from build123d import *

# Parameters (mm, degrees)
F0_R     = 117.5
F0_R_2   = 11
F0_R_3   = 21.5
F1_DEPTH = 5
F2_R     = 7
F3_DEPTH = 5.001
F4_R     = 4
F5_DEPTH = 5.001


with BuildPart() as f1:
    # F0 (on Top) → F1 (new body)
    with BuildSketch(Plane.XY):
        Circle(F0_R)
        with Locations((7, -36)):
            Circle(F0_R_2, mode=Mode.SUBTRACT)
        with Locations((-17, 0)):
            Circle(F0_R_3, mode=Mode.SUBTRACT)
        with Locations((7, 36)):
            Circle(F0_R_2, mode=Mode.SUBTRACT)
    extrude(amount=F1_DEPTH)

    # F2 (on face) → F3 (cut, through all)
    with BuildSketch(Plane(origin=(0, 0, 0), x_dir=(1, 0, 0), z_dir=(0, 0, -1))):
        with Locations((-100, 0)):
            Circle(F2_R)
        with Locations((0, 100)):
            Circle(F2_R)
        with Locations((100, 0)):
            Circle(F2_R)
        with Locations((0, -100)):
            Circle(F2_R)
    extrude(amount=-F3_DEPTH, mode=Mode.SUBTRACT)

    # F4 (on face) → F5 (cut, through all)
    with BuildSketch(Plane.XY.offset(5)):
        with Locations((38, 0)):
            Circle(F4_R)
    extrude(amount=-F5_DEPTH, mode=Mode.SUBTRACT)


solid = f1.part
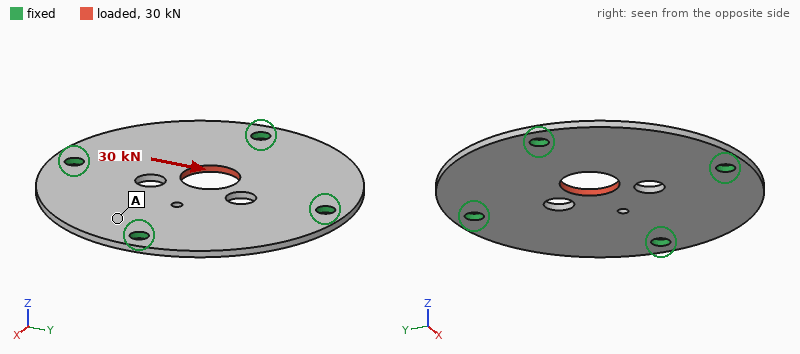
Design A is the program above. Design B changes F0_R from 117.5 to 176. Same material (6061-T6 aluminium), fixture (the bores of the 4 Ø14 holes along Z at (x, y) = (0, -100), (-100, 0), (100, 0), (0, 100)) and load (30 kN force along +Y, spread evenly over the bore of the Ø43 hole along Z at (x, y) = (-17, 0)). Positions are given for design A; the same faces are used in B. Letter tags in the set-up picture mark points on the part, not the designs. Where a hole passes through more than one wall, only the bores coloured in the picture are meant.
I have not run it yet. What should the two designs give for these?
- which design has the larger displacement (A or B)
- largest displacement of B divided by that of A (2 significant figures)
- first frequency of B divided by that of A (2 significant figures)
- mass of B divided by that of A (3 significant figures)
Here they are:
A
0.89
0.38
2.33
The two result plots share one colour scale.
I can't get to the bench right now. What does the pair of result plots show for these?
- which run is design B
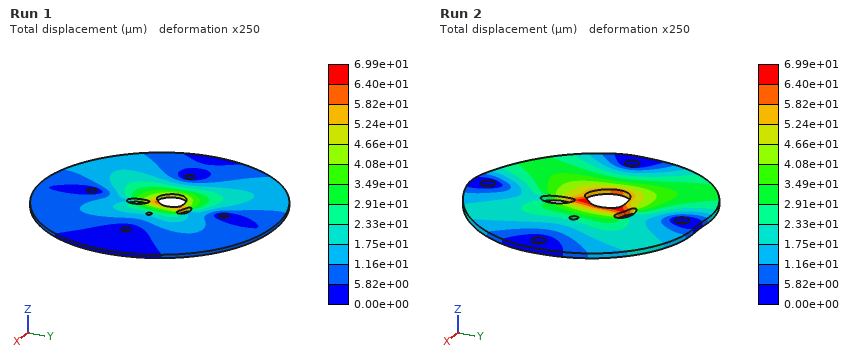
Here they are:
Run 1
